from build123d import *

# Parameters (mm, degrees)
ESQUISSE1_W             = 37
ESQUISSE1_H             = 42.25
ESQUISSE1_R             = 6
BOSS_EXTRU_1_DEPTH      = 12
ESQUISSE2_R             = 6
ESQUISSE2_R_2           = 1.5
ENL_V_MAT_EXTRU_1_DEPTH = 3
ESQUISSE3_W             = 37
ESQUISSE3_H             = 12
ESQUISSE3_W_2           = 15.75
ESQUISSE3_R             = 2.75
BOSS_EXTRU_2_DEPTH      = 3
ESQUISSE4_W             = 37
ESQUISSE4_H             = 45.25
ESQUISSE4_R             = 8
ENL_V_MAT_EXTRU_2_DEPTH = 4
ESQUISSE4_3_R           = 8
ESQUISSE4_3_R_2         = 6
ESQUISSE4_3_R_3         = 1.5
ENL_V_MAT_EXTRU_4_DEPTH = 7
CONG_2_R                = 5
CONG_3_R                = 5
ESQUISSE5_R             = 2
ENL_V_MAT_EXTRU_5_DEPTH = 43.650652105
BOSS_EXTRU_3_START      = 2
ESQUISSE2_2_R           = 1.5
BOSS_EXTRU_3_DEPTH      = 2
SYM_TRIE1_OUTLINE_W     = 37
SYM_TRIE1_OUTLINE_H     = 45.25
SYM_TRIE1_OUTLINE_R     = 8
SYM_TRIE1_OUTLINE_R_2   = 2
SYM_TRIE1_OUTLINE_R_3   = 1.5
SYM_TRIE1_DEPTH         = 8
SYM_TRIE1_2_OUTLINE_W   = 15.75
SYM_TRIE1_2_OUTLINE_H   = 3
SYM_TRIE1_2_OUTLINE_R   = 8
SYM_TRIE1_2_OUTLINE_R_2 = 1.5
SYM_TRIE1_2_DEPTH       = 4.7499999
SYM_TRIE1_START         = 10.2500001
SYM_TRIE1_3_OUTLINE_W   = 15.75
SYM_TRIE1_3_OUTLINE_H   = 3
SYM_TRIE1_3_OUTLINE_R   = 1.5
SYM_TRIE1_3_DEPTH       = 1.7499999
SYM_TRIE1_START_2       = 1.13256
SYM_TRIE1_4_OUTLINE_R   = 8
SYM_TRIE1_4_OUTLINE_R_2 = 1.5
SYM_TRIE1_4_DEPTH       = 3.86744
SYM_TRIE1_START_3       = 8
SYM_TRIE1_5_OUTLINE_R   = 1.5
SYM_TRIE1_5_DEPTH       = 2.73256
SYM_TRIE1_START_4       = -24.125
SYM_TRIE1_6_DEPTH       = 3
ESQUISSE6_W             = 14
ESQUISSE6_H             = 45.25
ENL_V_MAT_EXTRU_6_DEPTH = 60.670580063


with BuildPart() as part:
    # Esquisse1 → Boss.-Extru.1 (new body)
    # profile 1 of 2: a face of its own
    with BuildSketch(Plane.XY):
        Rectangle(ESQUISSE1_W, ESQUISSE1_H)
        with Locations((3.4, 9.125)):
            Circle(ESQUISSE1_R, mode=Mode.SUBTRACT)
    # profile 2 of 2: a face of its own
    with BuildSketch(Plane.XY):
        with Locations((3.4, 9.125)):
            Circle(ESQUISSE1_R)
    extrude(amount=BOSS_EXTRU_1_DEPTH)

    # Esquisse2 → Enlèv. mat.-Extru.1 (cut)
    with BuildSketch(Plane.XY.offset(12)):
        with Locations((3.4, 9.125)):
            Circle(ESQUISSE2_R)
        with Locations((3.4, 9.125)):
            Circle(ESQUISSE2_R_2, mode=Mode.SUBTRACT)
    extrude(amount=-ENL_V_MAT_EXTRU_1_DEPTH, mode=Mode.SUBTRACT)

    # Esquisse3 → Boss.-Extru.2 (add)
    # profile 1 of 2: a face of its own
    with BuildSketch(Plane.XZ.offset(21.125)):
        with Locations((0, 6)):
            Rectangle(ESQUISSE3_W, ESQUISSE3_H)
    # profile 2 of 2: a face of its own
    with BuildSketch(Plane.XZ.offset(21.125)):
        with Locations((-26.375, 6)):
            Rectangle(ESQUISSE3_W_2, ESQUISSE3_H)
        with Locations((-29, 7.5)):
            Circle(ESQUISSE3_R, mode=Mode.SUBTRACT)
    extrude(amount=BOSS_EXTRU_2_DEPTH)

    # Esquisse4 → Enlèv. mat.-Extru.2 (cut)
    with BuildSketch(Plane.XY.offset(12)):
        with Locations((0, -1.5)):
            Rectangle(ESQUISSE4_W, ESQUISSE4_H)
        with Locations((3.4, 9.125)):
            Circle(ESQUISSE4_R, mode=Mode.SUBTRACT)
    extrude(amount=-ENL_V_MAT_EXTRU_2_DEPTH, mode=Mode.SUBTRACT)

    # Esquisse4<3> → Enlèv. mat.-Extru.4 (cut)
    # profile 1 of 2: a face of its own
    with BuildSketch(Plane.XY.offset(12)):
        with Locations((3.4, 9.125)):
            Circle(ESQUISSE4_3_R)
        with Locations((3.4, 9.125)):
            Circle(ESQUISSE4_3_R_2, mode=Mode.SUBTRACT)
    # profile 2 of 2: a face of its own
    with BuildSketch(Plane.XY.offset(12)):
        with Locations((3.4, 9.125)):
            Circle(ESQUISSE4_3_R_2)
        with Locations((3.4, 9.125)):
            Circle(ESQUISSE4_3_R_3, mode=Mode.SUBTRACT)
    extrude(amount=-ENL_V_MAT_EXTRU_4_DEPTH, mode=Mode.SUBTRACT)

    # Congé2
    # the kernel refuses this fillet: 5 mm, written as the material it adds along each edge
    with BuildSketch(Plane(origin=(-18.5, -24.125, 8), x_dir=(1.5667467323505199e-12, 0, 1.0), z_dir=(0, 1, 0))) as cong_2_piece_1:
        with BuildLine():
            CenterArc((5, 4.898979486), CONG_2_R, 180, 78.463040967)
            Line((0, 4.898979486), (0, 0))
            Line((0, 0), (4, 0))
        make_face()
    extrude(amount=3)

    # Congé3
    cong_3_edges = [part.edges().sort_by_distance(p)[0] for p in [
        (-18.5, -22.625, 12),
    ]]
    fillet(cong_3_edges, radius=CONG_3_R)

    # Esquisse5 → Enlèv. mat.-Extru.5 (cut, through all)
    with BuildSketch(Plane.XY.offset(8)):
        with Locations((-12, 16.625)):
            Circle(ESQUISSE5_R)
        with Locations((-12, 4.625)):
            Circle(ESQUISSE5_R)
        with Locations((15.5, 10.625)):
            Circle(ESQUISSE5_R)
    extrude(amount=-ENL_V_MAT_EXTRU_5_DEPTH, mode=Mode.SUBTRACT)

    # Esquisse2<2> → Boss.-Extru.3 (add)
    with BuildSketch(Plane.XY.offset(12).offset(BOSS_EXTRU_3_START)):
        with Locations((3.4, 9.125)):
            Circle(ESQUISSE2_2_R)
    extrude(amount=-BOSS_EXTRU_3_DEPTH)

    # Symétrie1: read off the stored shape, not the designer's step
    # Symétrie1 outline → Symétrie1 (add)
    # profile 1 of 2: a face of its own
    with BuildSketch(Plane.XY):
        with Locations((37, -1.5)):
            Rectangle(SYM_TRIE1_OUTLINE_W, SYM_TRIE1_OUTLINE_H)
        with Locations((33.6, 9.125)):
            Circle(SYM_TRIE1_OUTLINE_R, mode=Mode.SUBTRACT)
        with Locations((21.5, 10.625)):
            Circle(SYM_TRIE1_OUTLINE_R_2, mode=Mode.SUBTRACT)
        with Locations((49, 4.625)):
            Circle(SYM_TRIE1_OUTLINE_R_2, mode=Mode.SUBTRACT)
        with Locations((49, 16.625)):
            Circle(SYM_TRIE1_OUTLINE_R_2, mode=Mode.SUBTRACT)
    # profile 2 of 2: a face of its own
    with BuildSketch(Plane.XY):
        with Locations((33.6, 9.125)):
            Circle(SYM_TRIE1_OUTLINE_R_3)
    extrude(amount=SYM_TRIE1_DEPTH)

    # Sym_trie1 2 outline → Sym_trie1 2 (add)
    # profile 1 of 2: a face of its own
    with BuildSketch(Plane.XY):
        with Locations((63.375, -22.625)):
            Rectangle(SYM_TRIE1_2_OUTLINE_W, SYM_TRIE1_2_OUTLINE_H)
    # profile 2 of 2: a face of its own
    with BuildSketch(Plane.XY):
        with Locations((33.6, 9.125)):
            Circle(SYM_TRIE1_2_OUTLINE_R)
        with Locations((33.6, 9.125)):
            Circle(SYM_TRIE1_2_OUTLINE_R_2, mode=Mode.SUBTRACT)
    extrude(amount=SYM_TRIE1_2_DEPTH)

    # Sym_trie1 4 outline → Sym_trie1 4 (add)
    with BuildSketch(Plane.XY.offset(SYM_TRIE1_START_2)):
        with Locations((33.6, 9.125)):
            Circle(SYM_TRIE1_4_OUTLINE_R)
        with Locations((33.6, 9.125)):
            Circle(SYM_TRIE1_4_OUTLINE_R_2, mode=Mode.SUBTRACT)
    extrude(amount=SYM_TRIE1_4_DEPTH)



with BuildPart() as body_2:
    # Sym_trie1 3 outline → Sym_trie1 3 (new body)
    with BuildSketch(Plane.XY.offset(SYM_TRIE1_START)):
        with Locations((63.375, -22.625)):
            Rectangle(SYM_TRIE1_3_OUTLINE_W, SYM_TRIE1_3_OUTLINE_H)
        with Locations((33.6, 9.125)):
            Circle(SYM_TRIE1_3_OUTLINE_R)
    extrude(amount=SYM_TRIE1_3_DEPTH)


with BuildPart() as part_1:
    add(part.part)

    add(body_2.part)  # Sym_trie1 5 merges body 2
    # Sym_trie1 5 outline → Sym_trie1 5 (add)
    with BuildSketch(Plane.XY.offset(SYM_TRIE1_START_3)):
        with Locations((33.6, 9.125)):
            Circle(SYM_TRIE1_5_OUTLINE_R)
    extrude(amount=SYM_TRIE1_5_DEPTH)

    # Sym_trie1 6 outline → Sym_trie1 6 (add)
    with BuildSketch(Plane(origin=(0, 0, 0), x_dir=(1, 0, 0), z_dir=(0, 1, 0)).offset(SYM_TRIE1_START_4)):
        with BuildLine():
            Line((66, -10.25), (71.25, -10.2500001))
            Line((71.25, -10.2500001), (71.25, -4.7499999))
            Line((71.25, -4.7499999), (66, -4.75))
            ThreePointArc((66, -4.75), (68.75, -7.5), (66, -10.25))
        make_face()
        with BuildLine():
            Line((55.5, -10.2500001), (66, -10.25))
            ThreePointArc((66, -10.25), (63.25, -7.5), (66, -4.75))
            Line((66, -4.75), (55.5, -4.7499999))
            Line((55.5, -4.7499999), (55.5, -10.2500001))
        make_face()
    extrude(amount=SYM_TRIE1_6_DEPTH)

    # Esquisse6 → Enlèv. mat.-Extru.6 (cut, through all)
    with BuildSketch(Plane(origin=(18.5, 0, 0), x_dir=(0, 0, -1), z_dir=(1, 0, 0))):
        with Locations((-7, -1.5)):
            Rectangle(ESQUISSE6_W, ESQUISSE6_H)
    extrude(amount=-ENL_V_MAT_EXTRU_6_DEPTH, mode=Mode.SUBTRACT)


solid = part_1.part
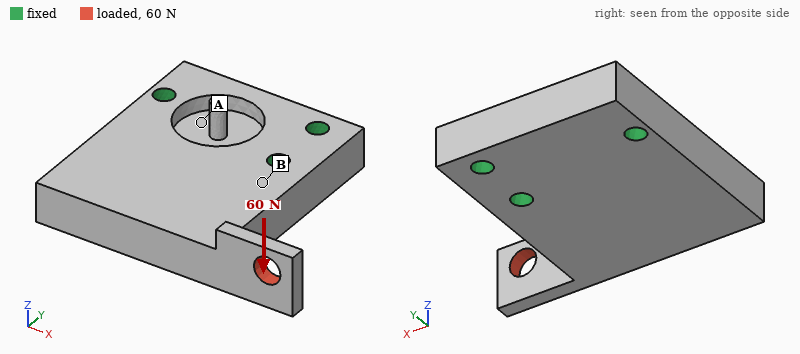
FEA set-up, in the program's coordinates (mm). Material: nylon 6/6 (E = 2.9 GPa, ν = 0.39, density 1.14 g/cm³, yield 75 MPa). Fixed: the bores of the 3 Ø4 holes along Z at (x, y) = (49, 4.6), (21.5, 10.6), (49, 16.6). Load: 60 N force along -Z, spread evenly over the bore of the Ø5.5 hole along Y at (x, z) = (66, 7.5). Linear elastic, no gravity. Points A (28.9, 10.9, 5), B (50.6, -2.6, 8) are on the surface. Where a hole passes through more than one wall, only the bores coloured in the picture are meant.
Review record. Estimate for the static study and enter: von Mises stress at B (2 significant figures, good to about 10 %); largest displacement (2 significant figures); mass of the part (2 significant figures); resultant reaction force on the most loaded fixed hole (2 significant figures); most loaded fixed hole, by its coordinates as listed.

6.9 MPa
0.65 mm
15 g
120 N
(49, 4.6)
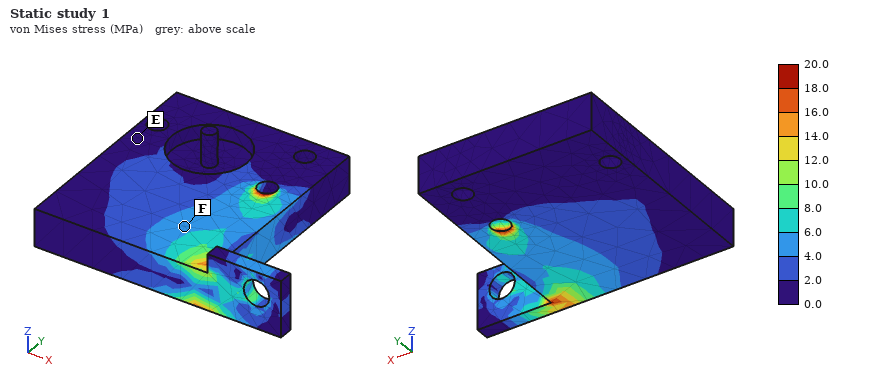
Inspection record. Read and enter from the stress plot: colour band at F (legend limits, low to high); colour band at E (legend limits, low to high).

4.0 to 6.0 MPa
0.0 to 2.0 MPa
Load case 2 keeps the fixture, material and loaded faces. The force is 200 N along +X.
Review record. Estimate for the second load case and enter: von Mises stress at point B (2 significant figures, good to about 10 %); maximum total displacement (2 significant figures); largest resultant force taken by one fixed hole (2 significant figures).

2.6 MPa
0.46 mm
220 N
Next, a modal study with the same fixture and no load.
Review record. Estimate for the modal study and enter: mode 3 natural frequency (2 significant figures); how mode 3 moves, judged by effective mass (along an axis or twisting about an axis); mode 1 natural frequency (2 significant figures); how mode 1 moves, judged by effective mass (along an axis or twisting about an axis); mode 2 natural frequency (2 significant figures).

2500 Hz
twisting about Y
1700 Hz
along Z
2400 Hz
